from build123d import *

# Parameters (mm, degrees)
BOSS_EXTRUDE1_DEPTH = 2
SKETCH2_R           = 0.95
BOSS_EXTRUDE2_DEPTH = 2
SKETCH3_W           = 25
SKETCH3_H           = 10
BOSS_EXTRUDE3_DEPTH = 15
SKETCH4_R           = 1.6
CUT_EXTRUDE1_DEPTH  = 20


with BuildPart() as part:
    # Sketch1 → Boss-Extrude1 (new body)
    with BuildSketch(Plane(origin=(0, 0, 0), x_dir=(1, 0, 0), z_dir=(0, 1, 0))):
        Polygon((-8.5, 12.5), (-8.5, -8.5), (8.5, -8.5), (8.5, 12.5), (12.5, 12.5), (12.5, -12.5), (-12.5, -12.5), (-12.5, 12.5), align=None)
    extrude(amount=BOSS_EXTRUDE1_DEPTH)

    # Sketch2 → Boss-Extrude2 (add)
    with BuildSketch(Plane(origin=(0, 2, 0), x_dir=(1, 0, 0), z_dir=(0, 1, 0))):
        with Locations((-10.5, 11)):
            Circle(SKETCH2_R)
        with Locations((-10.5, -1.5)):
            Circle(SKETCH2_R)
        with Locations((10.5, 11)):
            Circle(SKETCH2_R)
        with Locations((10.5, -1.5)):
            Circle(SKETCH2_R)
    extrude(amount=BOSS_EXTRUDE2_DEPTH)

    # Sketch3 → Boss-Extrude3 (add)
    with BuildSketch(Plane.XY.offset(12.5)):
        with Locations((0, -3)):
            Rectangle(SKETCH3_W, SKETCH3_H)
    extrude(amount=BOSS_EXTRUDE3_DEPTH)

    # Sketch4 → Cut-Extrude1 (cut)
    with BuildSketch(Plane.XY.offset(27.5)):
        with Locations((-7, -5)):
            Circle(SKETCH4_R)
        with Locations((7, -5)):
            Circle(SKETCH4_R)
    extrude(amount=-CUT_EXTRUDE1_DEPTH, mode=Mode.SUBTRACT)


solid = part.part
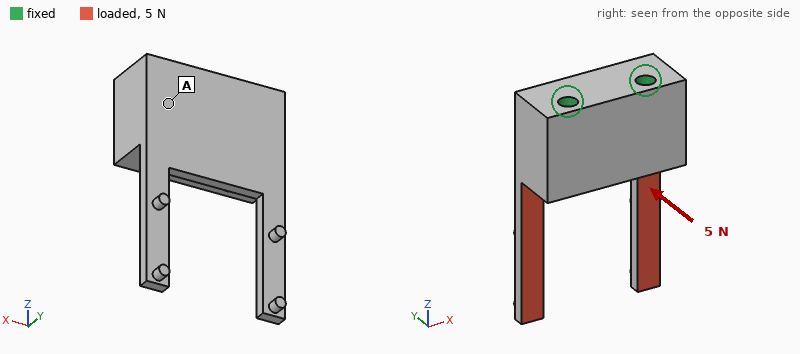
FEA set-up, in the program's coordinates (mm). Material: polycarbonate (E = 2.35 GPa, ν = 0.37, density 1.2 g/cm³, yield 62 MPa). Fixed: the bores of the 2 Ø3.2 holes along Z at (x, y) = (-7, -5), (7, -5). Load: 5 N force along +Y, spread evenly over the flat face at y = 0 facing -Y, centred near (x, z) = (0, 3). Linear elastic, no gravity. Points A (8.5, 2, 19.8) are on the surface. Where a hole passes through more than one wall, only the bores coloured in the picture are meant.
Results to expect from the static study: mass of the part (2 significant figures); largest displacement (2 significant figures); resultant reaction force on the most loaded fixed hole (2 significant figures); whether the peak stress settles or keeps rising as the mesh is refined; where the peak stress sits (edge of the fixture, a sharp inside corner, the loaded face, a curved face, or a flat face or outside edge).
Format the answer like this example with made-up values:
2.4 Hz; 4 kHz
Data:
4.9 g; 0.53 mm; 2.5 N; keeps rising; a sharp inside corner
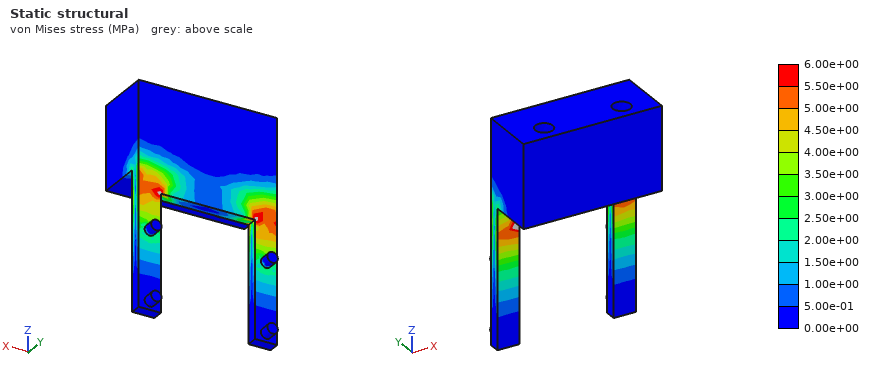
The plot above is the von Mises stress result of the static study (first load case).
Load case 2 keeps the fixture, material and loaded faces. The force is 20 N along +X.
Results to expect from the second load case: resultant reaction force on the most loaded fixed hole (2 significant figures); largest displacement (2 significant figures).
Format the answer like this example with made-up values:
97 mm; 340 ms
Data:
16 N; 0.47 mm
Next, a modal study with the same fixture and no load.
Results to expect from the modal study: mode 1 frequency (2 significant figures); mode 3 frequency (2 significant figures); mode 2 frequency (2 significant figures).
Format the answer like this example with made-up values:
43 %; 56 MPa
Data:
720 Hz; 1600 Hz; 720 Hz
